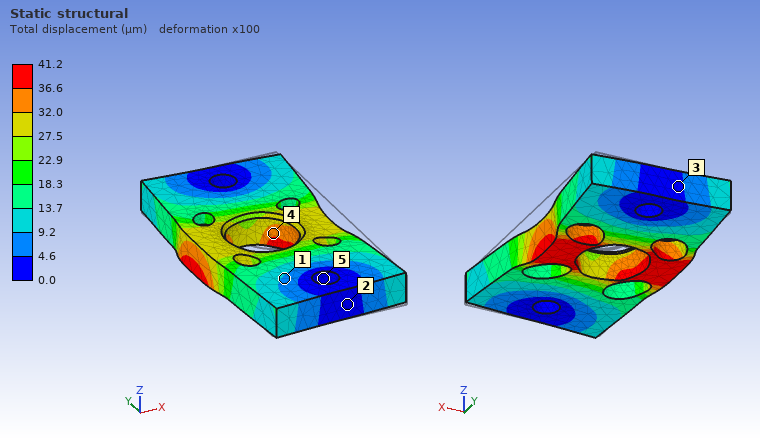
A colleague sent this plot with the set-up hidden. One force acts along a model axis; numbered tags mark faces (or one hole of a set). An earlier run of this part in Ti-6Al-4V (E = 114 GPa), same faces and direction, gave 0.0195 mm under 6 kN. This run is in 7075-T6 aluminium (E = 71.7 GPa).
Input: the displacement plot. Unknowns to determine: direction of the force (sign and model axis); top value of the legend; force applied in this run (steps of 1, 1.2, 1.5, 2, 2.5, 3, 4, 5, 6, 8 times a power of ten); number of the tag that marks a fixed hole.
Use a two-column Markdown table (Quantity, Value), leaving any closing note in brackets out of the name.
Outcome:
| Quantity | Value |
|---|---|
| direction of the force | -X |
| top value of the legend | 41.2 µm |
| force applied in this run | 8 kN |
| number of the tag that marks a fixed hole | 5 |
